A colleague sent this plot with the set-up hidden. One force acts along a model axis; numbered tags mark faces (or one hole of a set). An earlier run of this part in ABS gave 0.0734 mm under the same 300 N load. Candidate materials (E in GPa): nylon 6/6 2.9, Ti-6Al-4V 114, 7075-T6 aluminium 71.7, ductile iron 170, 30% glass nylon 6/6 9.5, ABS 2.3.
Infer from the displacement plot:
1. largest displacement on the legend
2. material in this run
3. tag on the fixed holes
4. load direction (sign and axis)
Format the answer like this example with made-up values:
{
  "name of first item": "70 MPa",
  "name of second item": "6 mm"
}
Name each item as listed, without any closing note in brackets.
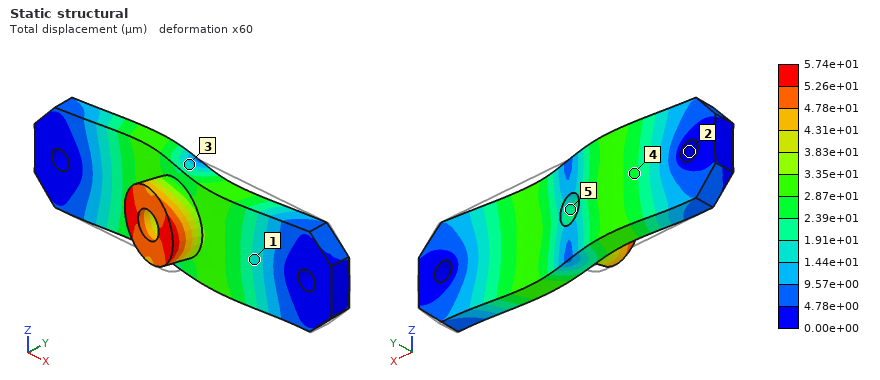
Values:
{
  "largest displacement on the legend": "5.74e+01 µm",
  "material in this run": "nylon 6/6",
  "tag on the fixed holes": "2",
  "load direction": "-X"
}
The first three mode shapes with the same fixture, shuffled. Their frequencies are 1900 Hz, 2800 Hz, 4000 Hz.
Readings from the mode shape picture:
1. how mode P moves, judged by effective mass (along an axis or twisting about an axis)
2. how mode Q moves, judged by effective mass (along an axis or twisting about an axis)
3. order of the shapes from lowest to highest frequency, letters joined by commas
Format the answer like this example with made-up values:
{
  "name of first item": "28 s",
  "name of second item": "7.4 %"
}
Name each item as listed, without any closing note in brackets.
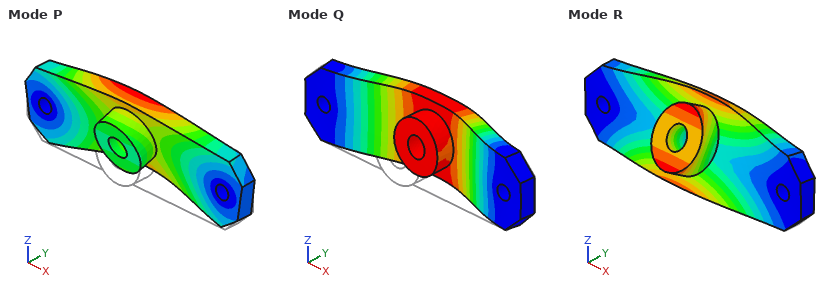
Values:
{
  "how mode P moves, judged by effective mass": "along Z",
  "how mode Q moves, judged by effective mass": "along Y",
  "order of the shapes from lowest to highest frequency, letters joined by commas": "Q, R, P"
}
